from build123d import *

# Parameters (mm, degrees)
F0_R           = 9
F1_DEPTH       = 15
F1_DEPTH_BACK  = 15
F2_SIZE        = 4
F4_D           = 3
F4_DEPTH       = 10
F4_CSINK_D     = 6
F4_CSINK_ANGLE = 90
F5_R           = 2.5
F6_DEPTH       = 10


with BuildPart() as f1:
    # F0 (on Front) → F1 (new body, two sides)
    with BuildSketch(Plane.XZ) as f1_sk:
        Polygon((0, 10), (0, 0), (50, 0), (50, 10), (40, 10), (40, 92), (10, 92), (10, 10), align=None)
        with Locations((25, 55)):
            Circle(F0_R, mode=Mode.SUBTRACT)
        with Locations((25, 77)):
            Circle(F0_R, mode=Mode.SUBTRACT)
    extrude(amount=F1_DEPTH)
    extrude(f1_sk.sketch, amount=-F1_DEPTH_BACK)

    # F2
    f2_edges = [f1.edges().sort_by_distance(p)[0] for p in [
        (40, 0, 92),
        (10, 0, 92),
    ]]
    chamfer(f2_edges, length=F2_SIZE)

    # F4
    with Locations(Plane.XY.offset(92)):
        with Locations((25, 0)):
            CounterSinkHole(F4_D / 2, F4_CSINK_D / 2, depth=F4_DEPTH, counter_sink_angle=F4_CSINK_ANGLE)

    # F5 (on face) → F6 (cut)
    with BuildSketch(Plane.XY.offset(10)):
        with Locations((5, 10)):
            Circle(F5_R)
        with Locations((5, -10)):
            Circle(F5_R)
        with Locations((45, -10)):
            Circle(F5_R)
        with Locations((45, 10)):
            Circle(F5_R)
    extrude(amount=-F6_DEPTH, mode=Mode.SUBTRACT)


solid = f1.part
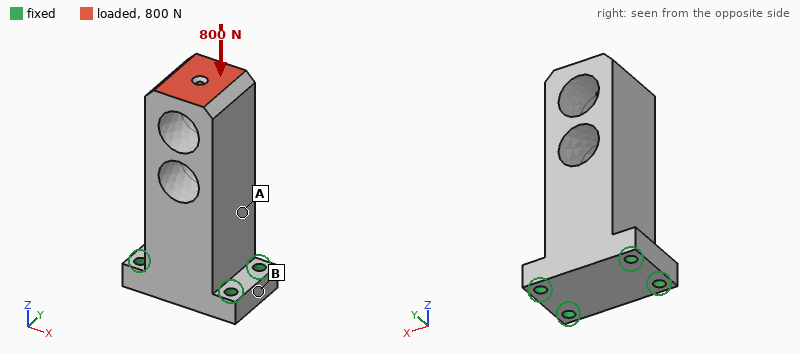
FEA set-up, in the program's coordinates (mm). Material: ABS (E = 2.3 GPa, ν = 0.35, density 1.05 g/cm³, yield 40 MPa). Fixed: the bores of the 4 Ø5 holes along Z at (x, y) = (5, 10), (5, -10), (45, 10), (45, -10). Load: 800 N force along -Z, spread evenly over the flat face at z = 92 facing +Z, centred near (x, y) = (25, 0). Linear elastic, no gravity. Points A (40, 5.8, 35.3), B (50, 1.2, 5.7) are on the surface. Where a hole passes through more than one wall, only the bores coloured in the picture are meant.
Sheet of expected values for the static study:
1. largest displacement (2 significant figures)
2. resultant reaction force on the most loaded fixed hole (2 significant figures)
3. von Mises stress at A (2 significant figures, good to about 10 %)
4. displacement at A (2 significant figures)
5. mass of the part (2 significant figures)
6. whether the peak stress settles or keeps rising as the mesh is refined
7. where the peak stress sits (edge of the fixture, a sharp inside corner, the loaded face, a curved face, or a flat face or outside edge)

0.11 mm
210 N
1.2 MPa
0.029 mm
76 g
keeps rising
edge of the fixture
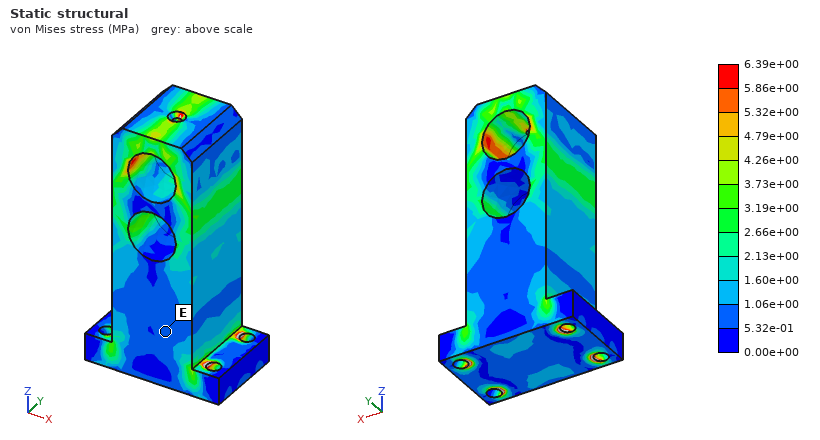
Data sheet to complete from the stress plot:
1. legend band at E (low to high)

5.32e-01 to 1.06e+00 MPa
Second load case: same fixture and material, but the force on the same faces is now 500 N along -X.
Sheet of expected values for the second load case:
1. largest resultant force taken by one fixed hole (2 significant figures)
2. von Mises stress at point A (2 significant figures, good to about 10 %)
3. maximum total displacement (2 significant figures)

650 N
7.1 MPa
1.2 mm
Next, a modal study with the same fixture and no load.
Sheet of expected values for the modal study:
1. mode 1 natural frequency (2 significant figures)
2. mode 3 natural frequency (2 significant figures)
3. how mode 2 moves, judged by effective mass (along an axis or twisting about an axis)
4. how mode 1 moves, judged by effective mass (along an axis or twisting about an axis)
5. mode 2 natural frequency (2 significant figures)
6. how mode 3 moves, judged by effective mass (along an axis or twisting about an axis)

700 Hz
2200 Hz
along X
along Y
870 Hz
twisting about Z
